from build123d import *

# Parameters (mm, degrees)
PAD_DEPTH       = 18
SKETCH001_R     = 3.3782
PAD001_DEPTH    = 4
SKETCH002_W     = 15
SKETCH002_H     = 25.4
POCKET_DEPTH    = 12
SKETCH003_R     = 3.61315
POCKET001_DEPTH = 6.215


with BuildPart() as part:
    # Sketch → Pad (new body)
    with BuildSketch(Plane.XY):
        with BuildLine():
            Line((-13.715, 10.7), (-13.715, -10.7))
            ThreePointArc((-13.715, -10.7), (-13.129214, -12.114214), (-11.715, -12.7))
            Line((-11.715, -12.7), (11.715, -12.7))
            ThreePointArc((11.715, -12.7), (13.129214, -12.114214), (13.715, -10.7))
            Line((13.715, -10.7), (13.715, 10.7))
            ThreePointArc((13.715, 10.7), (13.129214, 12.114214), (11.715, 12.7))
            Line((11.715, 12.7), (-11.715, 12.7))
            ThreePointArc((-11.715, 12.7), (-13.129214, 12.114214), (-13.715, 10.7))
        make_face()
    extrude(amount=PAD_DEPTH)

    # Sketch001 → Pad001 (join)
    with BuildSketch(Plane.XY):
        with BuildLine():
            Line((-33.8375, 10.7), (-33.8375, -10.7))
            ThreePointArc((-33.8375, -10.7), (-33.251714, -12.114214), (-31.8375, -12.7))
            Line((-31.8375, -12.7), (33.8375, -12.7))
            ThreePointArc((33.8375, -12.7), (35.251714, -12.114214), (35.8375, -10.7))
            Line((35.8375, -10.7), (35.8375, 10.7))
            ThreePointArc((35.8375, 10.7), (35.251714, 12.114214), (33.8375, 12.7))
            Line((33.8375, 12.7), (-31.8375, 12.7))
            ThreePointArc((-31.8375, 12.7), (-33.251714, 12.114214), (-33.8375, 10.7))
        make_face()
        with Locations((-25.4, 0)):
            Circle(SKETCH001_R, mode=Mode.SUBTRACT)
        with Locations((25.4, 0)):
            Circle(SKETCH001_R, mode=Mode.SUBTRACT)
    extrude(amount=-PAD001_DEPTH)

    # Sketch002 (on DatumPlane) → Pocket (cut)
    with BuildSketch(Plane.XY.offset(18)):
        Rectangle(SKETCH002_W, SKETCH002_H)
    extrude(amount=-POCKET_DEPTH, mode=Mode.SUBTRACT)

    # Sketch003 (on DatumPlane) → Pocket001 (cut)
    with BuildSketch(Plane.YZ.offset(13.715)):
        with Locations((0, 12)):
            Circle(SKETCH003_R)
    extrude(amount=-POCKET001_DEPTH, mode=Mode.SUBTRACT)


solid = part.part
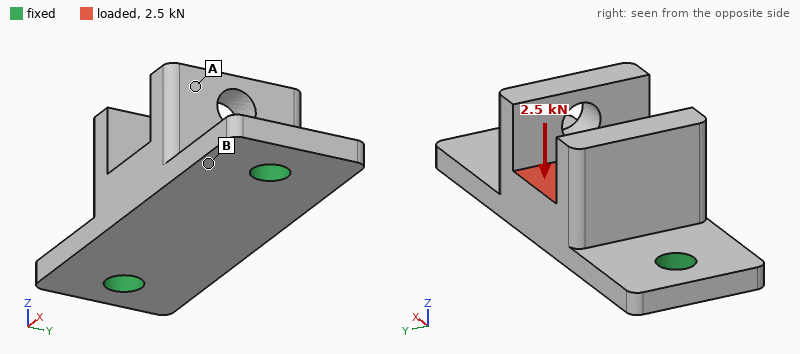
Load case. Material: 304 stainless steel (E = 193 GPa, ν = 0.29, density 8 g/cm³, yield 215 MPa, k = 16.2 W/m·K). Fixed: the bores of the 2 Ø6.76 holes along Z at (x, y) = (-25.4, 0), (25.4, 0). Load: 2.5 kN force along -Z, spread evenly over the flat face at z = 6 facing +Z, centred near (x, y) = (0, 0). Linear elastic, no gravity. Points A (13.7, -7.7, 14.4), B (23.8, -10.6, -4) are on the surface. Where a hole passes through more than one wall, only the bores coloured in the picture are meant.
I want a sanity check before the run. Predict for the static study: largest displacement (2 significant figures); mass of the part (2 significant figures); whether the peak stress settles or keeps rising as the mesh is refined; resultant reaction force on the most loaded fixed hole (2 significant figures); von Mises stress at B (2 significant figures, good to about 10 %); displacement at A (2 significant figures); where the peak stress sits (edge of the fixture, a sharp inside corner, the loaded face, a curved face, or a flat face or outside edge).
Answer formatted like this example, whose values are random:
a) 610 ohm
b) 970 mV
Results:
a) 15 µm
b) 120 g
c) keeps rising
d) 1.6 kN
e) 33 MPa
f) 12 µm
g) edge of the fixture
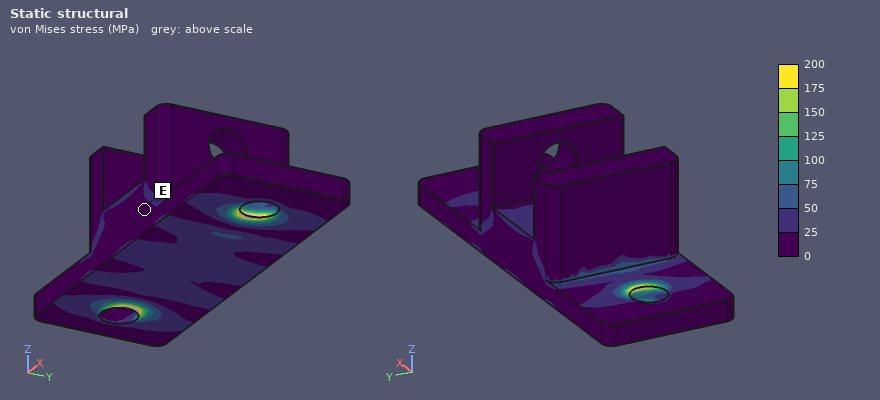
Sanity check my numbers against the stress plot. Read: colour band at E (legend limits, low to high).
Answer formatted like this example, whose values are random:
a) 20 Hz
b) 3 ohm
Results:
a) 0 to 25 MPa
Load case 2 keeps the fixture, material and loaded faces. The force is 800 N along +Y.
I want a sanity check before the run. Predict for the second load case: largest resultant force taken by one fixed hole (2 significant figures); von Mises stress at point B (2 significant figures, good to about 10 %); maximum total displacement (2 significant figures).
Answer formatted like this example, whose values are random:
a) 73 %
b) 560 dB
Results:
a) 400 N
b) 18 MPa
c) 17 µm
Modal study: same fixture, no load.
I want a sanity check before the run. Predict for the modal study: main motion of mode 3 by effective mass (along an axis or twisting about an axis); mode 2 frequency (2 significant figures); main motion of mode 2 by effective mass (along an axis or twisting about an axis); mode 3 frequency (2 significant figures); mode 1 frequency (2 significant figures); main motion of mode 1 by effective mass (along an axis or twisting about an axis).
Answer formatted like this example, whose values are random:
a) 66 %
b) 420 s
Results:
a) along X
b) 7500 Hz
c) along Z
d) 11 kHz
e) 4500 Hz
f) along Y
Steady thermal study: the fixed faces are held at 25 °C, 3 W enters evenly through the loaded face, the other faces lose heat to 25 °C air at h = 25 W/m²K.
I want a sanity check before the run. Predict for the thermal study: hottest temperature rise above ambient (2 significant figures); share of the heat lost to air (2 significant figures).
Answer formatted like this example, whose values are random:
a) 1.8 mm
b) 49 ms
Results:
a) 13 K
b) 33 %
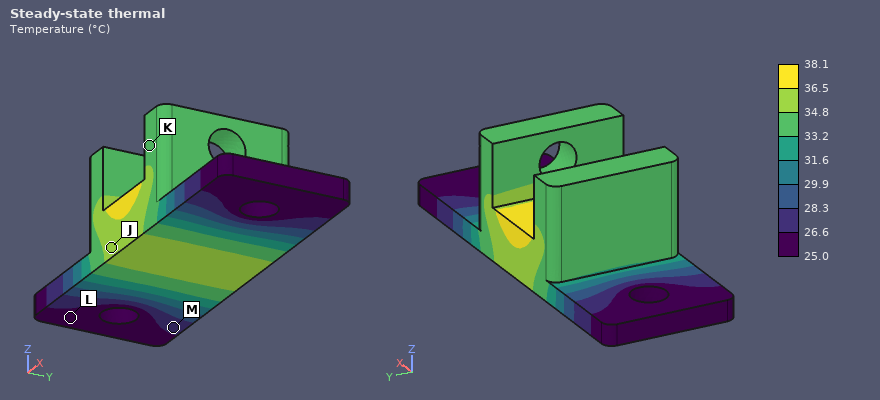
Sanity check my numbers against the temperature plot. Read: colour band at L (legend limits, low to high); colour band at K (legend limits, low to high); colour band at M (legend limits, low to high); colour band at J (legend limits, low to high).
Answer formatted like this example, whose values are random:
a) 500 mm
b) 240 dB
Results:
a) 25.0 to 26.6 °C
b) 33.2 to 34.8 °C
c) 26.6 to 28.3 °C
d) 34.8 to 36.5 °C
